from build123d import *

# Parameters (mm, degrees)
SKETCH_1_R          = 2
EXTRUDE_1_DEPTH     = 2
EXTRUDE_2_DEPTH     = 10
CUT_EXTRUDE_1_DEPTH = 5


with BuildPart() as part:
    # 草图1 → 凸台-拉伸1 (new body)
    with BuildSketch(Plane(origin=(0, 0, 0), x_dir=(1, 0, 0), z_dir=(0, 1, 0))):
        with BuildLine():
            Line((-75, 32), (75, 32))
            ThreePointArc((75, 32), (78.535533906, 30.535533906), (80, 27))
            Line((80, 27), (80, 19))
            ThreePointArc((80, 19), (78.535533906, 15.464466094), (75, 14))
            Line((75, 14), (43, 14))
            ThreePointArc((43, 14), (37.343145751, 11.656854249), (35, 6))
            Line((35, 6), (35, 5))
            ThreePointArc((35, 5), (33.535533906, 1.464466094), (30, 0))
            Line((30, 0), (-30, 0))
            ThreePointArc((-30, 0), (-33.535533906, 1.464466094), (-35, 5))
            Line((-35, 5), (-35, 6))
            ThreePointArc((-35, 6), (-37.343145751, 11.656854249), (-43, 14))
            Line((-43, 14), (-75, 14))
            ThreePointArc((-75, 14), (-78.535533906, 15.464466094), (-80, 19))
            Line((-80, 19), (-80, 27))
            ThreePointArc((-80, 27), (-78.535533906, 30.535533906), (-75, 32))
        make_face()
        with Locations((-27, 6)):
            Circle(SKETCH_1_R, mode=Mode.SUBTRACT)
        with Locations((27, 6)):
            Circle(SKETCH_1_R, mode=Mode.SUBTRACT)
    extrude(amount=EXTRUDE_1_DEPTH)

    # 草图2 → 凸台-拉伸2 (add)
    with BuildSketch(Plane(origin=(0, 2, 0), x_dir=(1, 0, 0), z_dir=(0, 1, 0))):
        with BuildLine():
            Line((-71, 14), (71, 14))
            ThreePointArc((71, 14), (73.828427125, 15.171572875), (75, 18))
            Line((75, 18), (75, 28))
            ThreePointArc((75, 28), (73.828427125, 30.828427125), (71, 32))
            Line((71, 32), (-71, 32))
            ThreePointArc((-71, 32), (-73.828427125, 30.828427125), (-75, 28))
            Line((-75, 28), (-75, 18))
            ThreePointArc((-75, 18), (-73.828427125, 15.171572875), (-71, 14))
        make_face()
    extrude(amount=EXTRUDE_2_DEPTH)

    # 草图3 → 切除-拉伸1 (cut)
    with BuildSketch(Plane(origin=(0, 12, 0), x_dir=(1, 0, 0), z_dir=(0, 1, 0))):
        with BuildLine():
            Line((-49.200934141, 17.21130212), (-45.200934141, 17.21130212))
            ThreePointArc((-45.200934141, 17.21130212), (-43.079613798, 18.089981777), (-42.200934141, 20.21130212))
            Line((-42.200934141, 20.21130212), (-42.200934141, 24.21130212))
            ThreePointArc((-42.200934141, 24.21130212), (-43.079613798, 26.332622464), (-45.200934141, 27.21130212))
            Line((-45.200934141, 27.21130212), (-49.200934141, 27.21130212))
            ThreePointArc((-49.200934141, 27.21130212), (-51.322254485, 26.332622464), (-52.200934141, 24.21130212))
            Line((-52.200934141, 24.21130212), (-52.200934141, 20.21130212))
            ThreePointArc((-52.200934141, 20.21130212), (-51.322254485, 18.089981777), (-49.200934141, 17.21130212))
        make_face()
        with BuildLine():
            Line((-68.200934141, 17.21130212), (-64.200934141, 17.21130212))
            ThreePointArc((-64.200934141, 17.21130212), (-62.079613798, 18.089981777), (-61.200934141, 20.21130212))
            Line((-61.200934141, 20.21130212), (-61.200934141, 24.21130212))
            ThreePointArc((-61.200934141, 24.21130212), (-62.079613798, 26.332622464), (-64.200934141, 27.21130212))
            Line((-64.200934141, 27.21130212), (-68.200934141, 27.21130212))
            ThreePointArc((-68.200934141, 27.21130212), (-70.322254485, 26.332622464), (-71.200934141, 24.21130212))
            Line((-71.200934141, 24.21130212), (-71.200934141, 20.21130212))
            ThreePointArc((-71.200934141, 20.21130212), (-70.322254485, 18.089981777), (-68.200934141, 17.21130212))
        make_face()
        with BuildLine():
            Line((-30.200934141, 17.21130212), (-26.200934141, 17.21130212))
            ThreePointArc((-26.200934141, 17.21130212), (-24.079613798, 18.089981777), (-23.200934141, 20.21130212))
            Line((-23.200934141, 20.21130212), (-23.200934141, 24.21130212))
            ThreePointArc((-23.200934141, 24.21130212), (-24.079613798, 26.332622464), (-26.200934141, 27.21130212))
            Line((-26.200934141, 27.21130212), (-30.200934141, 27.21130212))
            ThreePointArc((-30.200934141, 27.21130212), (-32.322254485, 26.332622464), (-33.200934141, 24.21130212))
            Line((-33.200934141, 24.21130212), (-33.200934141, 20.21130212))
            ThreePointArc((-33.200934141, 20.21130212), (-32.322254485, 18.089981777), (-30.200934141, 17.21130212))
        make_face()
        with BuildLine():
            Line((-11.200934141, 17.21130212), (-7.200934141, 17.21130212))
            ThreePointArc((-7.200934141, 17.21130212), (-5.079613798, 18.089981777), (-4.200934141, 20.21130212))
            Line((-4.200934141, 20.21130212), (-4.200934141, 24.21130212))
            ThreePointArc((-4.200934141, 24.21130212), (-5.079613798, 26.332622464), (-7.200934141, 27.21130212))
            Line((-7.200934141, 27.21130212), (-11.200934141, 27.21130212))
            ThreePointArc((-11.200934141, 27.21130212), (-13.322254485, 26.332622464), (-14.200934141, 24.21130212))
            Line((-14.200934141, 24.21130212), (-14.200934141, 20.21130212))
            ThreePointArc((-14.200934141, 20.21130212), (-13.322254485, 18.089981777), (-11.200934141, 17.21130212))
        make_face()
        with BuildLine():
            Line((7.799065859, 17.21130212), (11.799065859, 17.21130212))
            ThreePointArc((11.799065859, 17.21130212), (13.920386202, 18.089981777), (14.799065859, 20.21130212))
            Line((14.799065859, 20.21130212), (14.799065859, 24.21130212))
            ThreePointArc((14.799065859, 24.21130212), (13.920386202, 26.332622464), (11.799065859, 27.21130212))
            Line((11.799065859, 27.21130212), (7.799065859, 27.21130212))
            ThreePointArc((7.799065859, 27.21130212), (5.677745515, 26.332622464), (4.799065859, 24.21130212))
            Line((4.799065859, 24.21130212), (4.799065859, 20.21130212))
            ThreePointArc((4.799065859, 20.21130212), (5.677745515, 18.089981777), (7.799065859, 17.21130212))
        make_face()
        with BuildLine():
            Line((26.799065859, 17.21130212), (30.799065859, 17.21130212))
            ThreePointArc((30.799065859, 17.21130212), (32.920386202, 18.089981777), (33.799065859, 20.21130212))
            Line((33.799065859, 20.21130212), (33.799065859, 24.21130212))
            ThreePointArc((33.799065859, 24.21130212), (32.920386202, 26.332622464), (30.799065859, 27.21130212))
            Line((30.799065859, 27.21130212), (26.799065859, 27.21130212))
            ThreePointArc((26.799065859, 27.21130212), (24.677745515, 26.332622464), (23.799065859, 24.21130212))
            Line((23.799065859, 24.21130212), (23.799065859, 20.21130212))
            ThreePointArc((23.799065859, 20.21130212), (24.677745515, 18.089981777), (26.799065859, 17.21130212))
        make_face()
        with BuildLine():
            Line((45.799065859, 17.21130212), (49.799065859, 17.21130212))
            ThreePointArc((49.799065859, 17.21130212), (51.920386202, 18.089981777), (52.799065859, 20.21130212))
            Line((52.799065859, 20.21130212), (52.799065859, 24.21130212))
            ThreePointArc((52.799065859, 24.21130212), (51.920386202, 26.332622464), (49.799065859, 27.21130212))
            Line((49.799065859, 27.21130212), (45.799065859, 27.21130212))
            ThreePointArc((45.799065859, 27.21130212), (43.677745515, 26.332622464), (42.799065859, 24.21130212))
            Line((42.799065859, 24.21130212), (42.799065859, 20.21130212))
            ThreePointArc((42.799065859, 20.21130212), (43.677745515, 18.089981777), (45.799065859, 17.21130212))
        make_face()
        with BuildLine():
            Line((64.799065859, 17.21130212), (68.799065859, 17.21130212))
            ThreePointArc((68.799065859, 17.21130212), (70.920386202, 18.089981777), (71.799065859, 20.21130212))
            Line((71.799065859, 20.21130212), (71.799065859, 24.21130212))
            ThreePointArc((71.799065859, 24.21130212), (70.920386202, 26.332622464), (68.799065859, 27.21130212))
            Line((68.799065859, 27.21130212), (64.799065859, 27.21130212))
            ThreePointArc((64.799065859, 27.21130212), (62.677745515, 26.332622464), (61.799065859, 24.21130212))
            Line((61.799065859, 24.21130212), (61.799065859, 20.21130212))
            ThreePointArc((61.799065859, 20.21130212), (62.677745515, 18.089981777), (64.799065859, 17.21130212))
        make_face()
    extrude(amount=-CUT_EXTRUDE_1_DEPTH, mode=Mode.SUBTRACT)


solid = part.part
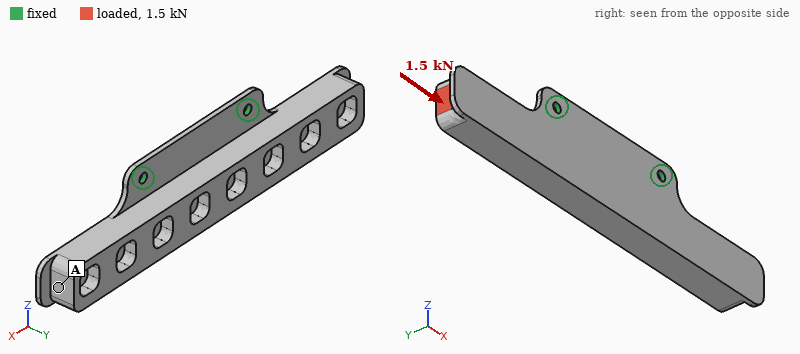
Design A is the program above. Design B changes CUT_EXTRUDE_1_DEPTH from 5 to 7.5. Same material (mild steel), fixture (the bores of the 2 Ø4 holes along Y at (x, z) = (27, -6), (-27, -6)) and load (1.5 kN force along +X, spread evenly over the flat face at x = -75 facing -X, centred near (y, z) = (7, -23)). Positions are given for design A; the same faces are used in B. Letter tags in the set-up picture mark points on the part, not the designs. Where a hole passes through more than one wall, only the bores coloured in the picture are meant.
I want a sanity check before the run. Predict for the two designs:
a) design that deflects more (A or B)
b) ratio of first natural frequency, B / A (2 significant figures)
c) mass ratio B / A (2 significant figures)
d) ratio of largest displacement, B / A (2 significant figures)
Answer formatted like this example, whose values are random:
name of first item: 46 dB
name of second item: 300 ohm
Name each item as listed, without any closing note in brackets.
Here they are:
design that deflects more: B
ratio of first natural frequency, B / A: 1.0
mass ratio B / A: 0.94
ratio of largest displacement, B / A: 1.1
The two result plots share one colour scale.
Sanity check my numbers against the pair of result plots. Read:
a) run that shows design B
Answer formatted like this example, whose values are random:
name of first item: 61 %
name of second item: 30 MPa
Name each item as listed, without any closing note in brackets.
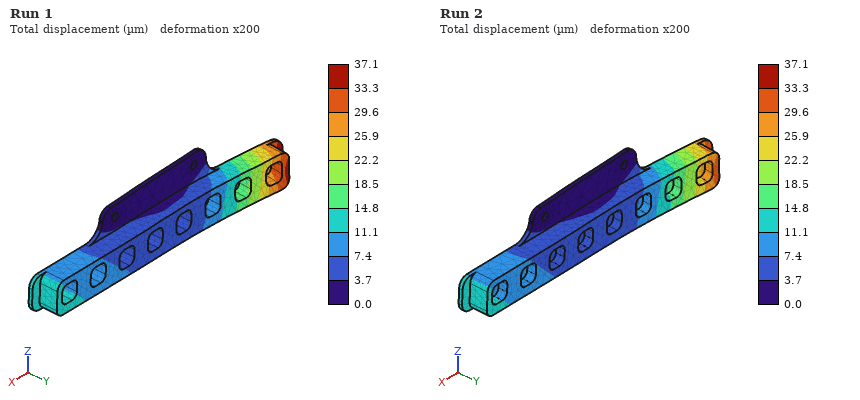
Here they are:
run that shows design B: Run 1
